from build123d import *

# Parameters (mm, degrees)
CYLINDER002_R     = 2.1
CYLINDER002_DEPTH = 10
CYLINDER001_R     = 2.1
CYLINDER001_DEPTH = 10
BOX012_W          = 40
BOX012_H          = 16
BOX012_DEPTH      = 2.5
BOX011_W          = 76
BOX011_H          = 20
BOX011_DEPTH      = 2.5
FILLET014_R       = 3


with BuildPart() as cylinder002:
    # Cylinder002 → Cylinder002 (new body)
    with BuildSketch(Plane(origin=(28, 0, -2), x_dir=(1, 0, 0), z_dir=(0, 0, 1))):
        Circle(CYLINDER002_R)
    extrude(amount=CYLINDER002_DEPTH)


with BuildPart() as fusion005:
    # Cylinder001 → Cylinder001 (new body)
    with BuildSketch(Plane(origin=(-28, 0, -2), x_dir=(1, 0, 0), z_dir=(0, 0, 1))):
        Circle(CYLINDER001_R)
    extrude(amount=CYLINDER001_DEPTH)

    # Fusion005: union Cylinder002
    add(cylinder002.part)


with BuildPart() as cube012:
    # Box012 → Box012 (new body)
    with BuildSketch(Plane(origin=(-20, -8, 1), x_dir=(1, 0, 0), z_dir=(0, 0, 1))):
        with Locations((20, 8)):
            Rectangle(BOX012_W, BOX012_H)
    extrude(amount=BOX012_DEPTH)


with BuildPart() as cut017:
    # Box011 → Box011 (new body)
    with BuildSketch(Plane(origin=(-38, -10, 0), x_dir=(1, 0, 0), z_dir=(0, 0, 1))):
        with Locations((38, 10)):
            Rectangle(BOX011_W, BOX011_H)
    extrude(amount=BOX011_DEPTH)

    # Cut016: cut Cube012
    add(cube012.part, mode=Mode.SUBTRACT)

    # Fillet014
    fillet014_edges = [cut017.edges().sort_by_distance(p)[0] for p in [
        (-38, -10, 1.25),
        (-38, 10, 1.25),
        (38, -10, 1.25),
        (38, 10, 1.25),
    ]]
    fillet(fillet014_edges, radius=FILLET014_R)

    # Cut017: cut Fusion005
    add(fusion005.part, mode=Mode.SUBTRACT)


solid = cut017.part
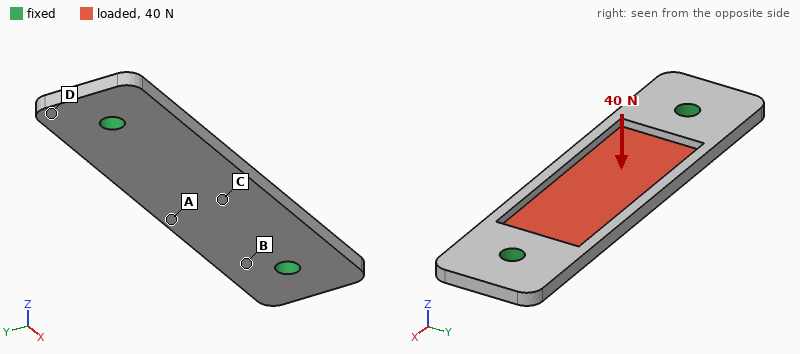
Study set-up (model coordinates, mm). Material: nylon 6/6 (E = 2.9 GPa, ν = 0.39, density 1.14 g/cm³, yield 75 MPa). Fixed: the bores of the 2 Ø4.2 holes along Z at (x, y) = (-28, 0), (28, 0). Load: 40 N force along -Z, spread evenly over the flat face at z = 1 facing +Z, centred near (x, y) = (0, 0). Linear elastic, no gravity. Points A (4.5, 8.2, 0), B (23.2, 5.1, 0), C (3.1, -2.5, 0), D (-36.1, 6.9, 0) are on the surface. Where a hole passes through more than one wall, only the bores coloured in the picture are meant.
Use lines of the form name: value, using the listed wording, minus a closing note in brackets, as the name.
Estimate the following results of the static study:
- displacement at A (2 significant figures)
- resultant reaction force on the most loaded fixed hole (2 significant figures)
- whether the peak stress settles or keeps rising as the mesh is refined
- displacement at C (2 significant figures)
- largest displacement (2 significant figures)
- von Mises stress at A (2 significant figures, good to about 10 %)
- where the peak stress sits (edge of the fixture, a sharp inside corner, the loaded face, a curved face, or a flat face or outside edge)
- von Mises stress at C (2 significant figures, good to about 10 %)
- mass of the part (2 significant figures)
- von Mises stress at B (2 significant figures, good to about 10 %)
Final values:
displacement at A: 0.52 mm
resultant reaction force on the most loaded fixed hole: 25 N
whether the peak stress settles or keeps rising as the mesh is refined: keeps rising
displacement at C: 0.62 mm
largest displacement: 0.64 mm
von Mises stress at A: 8.4 MPa
where the peak stress sits: edge of the fixture
von Mises stress at C: 10.0 MPa
mass of the part: 3.1 g
von Mises stress at B: 6.3 MPa
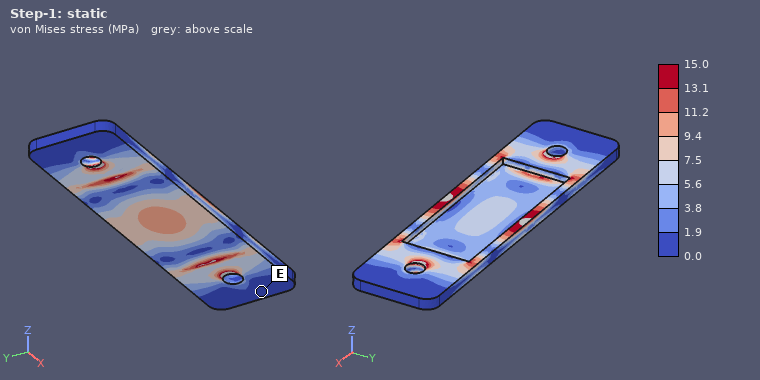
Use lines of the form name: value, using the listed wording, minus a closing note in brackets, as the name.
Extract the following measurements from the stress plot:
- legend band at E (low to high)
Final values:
legend band at E: 0.0 to 1.9 MPa
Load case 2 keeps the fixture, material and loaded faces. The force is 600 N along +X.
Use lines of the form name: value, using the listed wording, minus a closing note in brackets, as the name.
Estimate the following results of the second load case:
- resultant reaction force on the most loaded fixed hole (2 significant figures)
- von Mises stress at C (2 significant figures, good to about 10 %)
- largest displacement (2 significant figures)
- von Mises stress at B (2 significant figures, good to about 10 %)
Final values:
resultant reaction force on the most loaded fixed hole: 300 N
von Mises stress at C: 2.3 MPa
largest displacement: 0.10 mm
von Mises stress at B: 11 MPa
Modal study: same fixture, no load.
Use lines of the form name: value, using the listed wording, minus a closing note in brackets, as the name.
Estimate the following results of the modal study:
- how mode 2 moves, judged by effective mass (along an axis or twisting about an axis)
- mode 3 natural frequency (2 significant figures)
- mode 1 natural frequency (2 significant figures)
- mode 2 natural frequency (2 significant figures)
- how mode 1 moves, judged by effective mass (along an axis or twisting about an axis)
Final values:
how mode 2 moves, judged by effective mass: twisting about X
mode 3 natural frequency: 3300 Hz
mode 1 natural frequency: 1400 Hz
mode 2 natural frequency: 1800 Hz
how mode 1 moves, judged by effective mass: along Z
